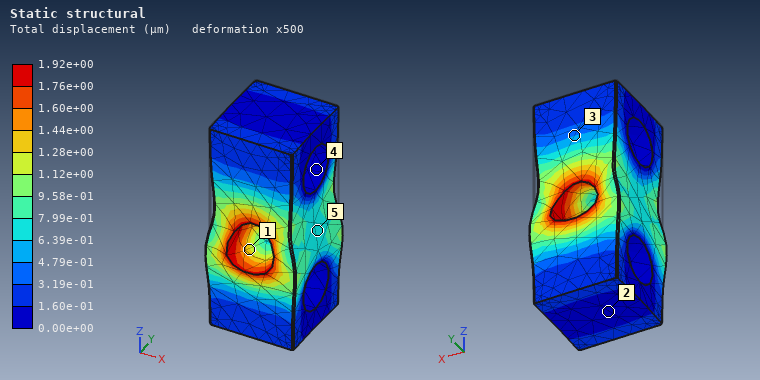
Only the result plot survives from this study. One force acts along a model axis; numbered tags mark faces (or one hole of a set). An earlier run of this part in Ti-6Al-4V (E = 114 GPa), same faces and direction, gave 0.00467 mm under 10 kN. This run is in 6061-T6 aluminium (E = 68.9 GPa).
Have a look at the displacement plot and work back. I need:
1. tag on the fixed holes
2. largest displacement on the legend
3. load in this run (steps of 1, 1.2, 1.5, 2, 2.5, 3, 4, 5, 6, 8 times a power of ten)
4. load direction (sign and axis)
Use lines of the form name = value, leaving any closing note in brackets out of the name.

tag on the fixed holes = 4
largest displacement on the legend = 1.92e+00 µm
load in this run = 2.5 kN
load direction = -Z
